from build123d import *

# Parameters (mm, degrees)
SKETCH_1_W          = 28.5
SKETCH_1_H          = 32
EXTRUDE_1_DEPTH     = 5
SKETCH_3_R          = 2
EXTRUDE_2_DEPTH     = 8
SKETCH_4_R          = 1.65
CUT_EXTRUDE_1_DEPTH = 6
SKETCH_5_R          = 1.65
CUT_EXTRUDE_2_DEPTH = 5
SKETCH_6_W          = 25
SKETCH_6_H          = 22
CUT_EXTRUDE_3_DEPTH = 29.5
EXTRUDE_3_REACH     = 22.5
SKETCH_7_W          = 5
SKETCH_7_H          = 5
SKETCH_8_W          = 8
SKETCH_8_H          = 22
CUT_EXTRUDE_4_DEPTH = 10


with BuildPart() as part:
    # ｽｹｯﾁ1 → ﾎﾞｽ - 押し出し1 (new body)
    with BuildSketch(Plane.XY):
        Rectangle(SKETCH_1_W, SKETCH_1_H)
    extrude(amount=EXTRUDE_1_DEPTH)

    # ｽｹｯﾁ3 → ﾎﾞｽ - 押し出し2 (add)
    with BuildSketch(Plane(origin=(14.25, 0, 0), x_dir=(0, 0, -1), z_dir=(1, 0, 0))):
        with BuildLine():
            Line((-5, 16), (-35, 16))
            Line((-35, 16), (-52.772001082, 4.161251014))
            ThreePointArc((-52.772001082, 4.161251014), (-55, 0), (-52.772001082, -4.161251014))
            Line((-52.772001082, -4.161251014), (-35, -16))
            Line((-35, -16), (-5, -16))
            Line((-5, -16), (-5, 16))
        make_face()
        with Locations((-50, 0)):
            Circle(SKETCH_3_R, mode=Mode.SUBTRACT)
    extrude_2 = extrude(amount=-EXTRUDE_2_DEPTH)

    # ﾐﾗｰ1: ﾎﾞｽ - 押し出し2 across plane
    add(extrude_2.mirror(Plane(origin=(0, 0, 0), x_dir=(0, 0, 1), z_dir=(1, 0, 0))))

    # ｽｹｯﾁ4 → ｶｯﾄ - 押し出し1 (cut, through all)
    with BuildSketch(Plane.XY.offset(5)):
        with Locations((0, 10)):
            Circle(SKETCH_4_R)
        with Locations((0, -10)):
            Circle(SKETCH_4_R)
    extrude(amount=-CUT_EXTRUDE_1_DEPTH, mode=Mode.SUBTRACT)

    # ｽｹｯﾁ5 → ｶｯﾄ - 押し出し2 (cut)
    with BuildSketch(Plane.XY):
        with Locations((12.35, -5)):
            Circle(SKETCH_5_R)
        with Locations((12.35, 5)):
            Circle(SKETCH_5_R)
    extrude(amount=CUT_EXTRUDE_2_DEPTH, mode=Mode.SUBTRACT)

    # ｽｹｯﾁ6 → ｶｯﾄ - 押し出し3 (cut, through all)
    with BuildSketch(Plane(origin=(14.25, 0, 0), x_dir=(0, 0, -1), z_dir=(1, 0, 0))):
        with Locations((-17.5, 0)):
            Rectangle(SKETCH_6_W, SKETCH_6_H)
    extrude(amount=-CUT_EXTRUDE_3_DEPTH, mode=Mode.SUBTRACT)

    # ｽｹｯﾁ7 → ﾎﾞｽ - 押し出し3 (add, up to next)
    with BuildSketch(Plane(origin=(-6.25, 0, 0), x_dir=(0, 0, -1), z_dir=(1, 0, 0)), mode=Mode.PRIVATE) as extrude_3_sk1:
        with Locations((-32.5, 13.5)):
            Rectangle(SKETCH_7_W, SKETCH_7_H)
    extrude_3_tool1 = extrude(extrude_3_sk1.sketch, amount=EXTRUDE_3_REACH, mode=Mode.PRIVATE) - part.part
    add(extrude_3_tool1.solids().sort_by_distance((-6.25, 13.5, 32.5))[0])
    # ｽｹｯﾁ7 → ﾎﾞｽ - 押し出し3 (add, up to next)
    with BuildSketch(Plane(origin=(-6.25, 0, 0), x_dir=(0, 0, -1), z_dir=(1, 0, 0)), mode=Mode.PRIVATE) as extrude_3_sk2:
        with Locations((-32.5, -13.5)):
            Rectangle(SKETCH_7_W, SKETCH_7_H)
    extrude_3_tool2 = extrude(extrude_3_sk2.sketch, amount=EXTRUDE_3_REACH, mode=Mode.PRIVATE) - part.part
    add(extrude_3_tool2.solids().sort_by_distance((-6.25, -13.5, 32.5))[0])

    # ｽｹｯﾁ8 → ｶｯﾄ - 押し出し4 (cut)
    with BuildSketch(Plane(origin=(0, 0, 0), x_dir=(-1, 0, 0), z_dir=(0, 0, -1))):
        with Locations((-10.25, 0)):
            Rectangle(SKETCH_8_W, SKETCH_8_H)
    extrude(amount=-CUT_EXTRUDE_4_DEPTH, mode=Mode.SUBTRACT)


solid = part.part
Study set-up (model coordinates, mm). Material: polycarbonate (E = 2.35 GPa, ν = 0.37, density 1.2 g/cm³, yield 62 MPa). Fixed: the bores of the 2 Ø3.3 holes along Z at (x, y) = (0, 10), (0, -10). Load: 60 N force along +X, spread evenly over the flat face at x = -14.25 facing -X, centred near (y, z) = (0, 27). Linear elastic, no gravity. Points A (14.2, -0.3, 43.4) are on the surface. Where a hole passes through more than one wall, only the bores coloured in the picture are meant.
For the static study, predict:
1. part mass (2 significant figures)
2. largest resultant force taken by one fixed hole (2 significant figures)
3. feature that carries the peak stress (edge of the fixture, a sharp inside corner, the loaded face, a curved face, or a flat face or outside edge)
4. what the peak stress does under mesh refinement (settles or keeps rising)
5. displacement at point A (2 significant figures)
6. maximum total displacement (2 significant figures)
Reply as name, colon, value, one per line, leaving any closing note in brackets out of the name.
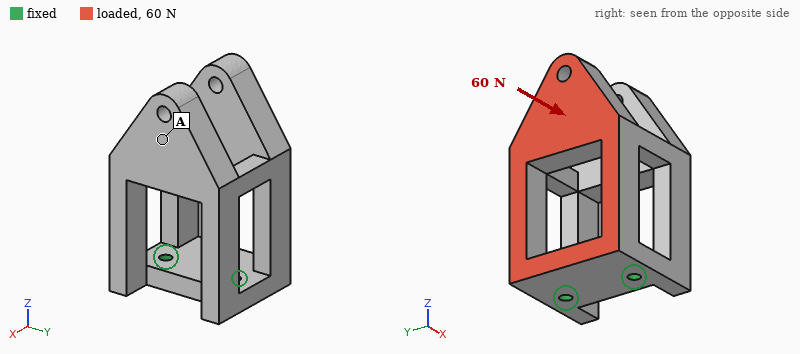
part mass: 20 g
largest resultant force taken by one fixed hole: 30 N
feature that carries the peak stress: edge of the fixture
what the peak stress does under mesh refinement: keeps rising
displacement at point A: 0.50 mm
maximum total displacement: 0.68 mm
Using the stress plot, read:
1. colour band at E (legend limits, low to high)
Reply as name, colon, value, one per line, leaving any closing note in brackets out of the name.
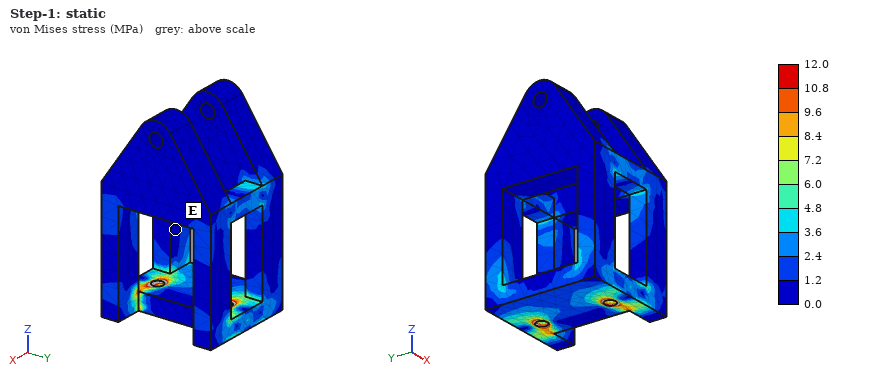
colour band at E: 0.0 to 1.2 MPa
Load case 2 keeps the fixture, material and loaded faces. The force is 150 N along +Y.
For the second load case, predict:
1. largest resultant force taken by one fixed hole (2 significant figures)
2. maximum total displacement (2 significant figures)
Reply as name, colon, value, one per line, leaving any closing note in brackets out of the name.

largest resultant force taken by one fixed hole: 180 N
maximum total displacement: 0.84 mm
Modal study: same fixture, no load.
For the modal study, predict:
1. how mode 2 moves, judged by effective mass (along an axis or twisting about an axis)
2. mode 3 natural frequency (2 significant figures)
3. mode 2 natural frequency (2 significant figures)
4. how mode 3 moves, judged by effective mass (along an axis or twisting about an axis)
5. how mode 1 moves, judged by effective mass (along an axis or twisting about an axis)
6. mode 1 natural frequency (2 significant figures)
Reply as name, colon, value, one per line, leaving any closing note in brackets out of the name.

how mode 2 moves, judged by effective mass: along Y
mode 3 natural frequency: 1100 Hz
mode 2 natural frequency: 580 Hz
how mode 3 moves, judged by effective mass: twisting about Z
how mode 1 moves, judged by effective mass: along X
mode 1 natural frequency: 430 Hz
